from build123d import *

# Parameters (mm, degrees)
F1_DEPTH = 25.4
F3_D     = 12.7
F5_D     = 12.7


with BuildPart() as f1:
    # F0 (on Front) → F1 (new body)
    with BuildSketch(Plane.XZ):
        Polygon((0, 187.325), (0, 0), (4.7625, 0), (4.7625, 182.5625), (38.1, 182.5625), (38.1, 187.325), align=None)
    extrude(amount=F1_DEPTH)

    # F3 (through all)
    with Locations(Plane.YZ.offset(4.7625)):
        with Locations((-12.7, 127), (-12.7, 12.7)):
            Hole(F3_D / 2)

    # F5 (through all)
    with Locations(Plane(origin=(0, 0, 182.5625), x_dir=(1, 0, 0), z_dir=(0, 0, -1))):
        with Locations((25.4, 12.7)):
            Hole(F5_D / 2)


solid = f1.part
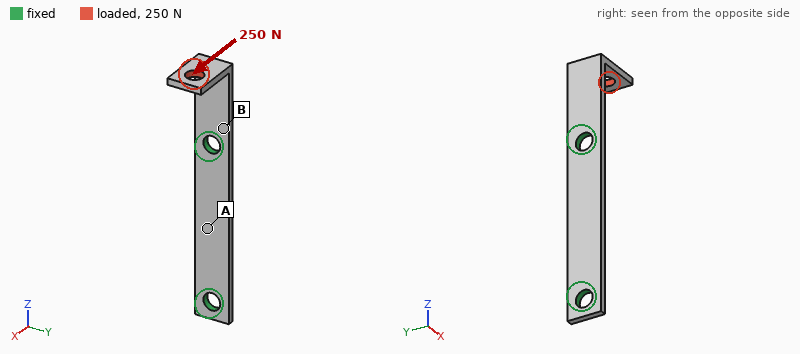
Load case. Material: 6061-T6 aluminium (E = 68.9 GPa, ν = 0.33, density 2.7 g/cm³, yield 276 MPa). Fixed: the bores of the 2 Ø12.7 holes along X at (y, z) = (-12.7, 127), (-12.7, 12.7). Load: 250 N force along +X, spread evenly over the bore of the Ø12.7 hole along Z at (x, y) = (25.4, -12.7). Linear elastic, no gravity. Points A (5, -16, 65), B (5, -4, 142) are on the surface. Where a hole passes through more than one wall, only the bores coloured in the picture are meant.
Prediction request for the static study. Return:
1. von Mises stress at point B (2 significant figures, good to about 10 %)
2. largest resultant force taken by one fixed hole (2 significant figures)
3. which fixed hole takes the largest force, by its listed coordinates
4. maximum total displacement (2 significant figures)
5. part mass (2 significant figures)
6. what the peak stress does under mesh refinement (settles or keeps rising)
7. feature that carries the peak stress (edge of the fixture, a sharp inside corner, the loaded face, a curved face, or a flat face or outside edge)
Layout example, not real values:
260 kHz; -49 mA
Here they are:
110 MPa; 250 N; (-12.7, 127); 1.1 mm; 67 g; keeps rising; edge of the fixture
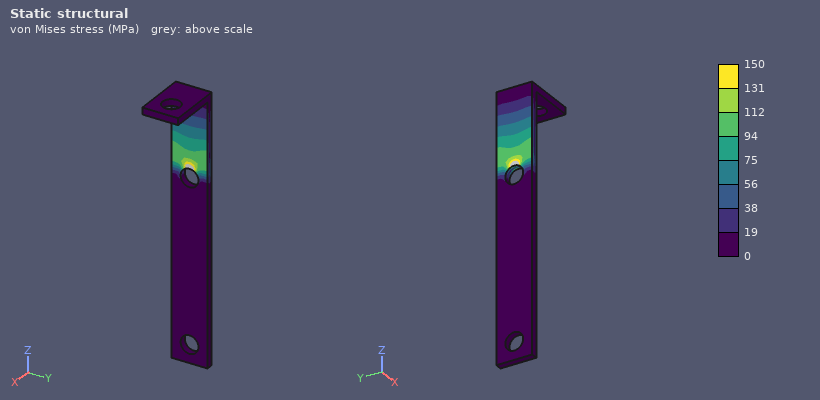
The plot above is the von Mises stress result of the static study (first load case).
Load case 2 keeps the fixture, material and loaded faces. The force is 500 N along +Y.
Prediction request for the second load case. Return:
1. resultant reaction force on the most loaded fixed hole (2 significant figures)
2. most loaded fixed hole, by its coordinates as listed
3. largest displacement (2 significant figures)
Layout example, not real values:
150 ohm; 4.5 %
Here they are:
530 N; (-12.7, 127); 1.1 mm
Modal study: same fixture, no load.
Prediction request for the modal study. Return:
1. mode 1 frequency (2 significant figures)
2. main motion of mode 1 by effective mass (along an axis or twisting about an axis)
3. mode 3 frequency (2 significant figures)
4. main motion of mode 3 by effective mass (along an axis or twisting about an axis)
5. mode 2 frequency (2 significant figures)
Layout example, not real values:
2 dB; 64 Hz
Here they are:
680 Hz; along X; 2300 Hz; along X; 1400 Hz
